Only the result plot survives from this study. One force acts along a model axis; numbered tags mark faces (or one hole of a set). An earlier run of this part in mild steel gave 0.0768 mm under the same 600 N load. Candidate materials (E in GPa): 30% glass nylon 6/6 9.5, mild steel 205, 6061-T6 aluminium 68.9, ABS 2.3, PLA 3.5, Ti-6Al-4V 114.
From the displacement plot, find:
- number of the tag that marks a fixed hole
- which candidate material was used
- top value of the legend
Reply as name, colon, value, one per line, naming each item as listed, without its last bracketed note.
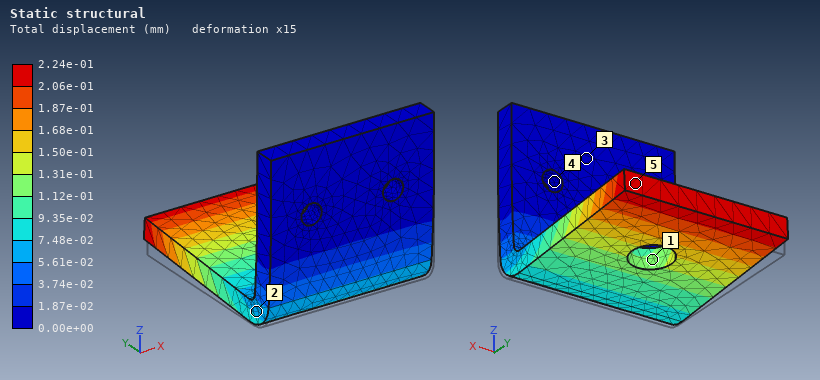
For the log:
number of the tag that marks a fixed hole: 4
which candidate material was used: 6061-T6 aluminium
top value of the legend: 2.24e-01 mm
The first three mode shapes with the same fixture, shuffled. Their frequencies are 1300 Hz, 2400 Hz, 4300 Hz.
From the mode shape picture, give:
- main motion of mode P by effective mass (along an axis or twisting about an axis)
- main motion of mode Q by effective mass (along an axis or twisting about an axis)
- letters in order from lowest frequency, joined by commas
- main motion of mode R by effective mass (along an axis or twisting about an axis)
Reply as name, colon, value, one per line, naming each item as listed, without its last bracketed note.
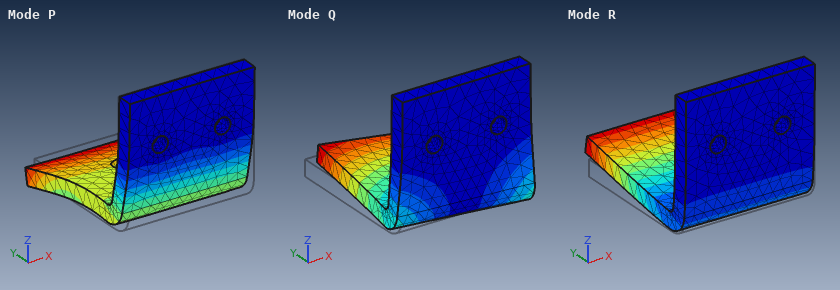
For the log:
main motion of mode P by effective mass: along Y
main motion of mode Q by effective mass: along X
letters in order from lowest frequency, joined by commas: R, Q, P
main motion of mode R by effective mass: along Z
